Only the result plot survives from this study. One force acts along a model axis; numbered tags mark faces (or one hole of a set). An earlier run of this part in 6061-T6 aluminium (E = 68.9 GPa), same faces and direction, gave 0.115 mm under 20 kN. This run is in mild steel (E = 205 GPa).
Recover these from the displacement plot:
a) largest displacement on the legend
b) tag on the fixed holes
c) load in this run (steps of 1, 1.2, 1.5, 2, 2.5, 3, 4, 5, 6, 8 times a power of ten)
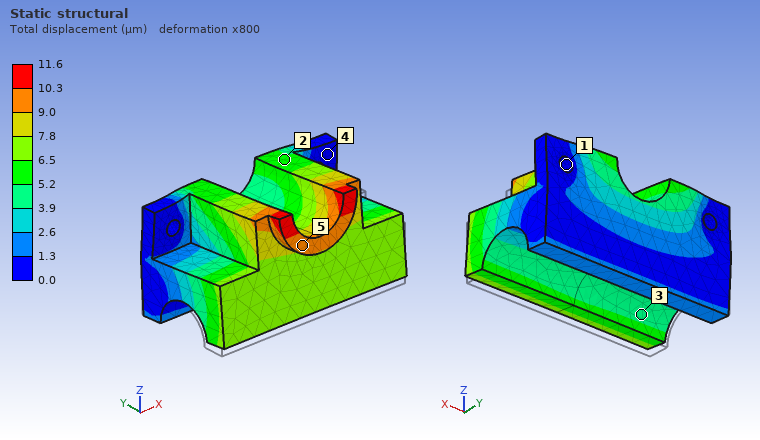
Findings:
11.6 µm
1
6 kN
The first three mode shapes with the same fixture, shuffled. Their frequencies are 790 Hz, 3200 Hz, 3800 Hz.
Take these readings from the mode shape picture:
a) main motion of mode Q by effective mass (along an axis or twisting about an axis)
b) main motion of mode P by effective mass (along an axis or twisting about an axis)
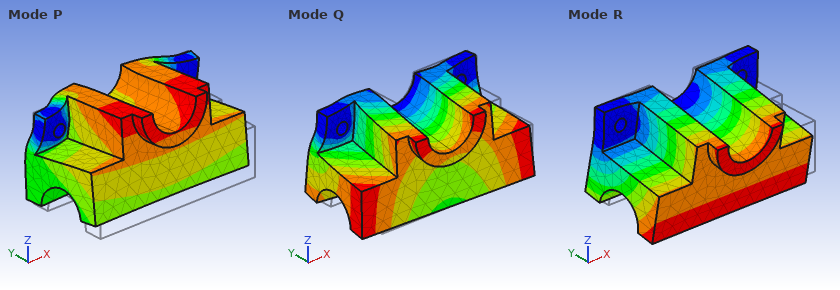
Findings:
along X
along Y
